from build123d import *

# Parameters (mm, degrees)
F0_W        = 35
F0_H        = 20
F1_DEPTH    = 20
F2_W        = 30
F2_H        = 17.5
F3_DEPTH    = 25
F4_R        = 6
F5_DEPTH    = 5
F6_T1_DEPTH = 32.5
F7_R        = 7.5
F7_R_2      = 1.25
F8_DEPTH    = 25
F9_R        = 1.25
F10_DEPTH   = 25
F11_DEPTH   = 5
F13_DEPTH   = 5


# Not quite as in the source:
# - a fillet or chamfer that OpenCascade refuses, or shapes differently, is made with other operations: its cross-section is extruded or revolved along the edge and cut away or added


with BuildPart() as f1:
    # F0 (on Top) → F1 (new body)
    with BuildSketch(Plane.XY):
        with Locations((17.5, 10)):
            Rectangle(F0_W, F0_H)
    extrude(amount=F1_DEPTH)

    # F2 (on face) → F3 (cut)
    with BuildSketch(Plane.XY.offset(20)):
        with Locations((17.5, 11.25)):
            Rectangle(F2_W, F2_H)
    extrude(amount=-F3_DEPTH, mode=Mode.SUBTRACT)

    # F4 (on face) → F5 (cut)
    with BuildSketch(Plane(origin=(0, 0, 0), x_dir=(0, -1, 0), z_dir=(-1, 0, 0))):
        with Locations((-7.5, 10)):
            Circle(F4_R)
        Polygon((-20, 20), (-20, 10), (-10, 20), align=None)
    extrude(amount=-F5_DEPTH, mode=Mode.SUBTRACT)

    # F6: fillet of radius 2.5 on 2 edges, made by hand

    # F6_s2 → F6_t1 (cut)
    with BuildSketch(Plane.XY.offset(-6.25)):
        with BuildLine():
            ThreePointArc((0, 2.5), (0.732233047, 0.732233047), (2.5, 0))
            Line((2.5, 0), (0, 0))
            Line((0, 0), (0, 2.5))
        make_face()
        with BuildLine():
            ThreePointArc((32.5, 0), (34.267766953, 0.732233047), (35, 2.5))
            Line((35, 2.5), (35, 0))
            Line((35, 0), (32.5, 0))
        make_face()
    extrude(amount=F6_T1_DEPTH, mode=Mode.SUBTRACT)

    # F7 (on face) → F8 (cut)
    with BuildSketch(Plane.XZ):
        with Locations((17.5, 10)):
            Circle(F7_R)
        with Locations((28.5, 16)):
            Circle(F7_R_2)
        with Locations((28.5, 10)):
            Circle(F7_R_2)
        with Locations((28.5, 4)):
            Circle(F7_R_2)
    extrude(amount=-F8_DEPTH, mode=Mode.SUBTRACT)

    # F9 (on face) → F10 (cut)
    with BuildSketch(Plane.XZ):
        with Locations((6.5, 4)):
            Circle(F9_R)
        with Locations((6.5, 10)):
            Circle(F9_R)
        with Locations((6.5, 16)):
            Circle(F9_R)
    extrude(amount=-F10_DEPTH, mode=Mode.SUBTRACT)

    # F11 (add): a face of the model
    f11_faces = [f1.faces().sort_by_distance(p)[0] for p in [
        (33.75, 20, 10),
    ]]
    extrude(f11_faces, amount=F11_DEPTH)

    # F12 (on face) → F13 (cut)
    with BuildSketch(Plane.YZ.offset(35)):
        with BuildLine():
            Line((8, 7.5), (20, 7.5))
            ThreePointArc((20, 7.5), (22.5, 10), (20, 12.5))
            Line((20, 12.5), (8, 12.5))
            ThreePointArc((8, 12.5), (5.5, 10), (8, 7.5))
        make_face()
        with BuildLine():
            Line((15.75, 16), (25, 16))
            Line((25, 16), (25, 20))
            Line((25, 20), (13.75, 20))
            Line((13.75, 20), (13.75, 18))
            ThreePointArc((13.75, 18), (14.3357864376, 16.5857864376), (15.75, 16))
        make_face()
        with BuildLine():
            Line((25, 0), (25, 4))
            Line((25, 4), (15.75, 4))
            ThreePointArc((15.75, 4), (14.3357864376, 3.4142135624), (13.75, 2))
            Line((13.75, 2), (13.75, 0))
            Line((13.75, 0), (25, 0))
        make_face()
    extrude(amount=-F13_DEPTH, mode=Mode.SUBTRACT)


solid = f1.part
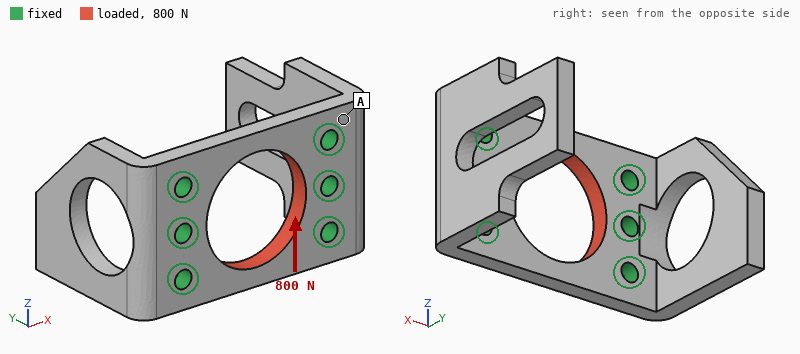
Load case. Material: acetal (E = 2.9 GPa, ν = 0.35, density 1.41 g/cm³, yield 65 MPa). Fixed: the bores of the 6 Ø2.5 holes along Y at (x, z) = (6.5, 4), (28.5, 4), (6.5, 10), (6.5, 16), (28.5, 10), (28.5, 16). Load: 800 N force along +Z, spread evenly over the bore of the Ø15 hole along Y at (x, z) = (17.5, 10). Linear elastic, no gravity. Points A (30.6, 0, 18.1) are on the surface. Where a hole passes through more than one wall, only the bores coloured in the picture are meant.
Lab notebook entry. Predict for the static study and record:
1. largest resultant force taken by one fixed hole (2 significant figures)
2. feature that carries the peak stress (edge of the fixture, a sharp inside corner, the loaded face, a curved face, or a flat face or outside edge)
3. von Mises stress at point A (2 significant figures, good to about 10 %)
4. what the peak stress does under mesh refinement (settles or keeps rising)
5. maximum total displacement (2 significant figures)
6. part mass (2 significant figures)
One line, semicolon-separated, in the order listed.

180 N; edge of the fixture; 4.5 MPa; keeps rising; 0.15 mm; 3.3 g
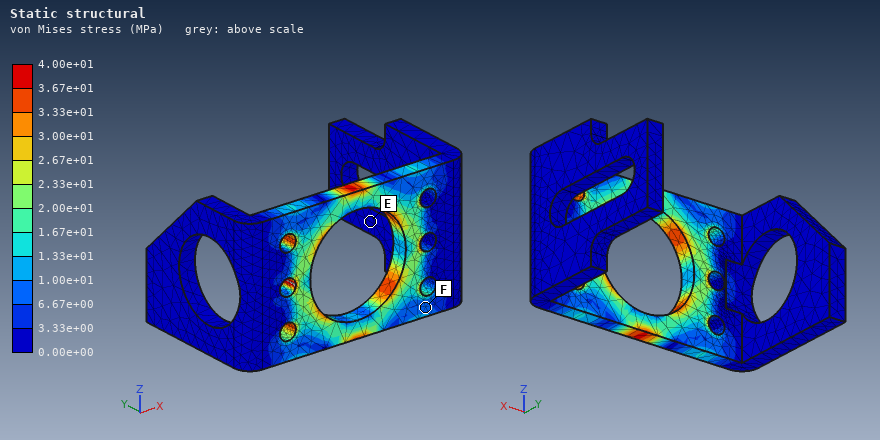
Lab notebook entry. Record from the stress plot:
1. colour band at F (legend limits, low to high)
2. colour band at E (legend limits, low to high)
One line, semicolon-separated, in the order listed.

6.67e+00 to 1.00e+01 MPa; 0.00e+00 to 3.33e+00 MPa
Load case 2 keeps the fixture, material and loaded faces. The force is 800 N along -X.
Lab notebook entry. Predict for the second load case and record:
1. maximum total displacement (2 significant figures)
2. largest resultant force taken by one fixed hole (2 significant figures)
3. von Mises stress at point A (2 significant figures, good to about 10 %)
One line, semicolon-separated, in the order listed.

37 µm; 160 N; 3.1 MPa
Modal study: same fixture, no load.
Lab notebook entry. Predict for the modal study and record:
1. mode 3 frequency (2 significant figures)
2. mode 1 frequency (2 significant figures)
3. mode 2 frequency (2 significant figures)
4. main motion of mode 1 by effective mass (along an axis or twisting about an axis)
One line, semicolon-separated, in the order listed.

2700 Hz; 1100 Hz; 1100 Hz; along X
